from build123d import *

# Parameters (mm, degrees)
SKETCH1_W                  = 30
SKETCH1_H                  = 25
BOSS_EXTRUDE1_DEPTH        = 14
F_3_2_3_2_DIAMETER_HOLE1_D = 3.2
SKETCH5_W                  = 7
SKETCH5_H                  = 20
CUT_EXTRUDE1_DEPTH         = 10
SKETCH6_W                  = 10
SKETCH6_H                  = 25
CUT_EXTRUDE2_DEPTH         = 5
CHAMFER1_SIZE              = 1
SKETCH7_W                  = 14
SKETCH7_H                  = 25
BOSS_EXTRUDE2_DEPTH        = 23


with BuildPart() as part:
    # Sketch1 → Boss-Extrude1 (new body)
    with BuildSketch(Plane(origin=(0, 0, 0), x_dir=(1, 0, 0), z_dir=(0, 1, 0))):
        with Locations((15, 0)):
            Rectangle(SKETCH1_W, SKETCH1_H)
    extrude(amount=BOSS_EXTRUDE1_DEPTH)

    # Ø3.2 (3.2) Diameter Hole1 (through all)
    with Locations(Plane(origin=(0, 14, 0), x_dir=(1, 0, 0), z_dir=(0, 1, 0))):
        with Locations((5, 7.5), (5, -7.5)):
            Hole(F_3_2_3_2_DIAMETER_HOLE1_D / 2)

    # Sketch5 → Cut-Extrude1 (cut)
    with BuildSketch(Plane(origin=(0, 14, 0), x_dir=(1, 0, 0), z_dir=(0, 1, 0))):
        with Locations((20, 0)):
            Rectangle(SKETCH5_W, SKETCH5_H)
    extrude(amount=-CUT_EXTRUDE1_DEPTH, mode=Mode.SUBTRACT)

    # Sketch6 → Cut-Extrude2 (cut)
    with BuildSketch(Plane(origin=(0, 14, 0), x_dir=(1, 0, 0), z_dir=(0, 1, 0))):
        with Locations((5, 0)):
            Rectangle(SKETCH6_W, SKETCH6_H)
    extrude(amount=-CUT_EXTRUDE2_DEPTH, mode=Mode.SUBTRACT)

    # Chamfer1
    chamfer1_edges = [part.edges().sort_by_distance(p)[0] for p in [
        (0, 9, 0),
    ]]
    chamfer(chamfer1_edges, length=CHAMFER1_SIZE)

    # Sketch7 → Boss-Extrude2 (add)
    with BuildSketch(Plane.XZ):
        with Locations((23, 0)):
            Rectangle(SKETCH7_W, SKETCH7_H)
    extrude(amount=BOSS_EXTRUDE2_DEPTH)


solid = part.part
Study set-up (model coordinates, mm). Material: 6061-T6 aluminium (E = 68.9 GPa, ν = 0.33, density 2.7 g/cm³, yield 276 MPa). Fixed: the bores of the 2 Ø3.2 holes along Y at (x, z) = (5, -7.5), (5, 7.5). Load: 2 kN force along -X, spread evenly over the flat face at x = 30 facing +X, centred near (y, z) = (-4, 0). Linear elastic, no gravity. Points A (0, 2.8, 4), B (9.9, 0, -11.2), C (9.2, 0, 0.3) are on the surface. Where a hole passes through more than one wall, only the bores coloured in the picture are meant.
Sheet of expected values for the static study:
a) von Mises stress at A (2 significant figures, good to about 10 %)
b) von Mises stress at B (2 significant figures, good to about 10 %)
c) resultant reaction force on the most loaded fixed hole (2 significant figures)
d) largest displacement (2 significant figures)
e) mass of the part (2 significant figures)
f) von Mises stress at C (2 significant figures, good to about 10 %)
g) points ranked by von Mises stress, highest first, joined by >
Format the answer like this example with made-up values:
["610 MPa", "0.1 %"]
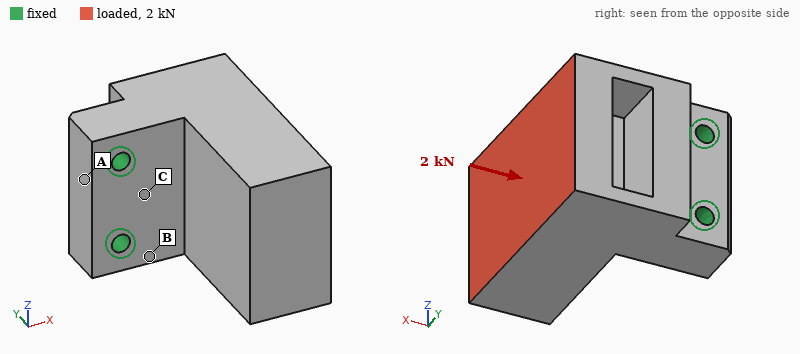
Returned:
["15 MPa", "56 MPa", "1.0 kN", "100 µm", "43 g", "38 MPa", "B > C > A"]
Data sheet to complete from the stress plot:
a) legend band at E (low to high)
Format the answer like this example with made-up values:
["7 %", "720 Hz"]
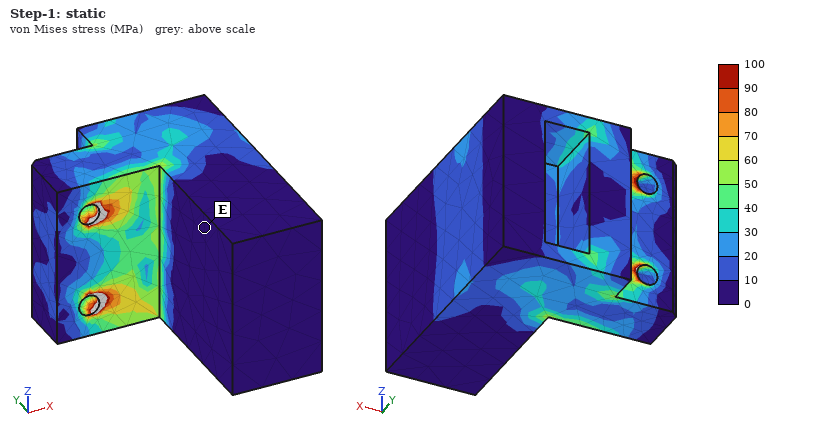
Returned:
["0 to 10 MPa"]
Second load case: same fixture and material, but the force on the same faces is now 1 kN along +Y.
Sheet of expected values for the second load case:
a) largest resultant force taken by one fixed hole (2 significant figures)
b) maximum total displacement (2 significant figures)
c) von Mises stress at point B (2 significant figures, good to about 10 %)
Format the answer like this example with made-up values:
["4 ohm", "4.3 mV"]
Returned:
["510 N", "0.10 mm", "54 MPa"]
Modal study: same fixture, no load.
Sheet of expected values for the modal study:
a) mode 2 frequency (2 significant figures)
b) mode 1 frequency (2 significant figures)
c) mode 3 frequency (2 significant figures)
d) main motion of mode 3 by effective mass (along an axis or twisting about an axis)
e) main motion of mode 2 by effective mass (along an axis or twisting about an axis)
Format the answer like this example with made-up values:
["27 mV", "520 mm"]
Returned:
["6300 Hz", "3700 Hz", "11 kHz", "along Z", "along Z"]
